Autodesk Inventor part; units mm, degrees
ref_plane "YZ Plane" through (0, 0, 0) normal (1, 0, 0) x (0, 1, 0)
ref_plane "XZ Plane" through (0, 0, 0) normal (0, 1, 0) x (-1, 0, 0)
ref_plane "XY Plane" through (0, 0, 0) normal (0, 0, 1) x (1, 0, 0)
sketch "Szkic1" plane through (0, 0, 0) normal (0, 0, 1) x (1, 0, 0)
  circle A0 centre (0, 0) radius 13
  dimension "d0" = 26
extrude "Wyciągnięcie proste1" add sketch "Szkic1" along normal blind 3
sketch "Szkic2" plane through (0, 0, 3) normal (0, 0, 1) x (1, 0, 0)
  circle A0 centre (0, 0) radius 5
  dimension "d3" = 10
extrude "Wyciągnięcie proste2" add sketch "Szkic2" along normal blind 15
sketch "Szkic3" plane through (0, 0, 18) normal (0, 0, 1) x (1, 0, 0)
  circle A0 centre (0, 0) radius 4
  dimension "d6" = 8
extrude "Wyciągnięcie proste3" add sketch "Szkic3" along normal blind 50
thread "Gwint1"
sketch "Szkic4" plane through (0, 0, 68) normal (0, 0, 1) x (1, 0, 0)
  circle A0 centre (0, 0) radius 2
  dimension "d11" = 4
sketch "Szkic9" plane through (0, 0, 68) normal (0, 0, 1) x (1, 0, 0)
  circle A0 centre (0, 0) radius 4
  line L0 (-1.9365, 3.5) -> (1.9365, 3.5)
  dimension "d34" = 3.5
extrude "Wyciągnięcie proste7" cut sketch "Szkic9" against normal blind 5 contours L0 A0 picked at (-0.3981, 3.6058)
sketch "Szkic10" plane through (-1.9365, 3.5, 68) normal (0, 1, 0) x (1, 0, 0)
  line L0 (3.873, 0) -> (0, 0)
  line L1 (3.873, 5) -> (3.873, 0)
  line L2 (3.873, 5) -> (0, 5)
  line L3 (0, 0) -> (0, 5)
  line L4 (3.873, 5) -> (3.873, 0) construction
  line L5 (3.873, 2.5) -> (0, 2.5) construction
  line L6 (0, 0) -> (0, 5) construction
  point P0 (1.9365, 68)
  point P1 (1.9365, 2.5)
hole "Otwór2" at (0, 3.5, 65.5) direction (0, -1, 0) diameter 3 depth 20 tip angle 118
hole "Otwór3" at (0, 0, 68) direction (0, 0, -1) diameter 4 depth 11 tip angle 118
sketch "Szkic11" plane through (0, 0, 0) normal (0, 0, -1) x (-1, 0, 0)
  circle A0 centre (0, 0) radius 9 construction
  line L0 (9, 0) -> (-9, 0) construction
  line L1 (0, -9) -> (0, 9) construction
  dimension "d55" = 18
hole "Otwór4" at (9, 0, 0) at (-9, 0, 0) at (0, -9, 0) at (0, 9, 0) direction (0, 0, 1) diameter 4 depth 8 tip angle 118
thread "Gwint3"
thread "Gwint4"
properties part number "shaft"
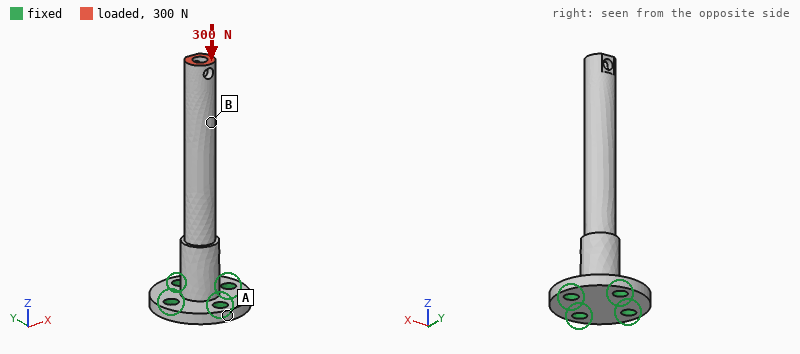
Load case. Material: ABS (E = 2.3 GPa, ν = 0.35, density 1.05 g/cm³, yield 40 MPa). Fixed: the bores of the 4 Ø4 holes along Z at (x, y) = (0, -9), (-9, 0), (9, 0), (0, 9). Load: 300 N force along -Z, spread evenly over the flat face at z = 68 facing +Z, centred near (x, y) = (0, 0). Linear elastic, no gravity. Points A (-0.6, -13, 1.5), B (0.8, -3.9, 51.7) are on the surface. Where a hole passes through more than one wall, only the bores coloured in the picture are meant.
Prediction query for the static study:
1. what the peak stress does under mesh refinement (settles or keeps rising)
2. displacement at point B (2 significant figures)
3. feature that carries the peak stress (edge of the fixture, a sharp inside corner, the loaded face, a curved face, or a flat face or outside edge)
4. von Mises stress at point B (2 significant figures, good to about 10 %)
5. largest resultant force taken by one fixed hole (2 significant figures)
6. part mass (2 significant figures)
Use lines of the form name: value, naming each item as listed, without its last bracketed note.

what the peak stress does under mesh refinement: keeps rising
displacement at point B: 0.17 mm
feature that carries the peak stress: a sharp inside corner
von Mises stress at point B: 6.9 MPa
largest resultant force taken by one fixed hole: 82 N
part mass: 5.2 g
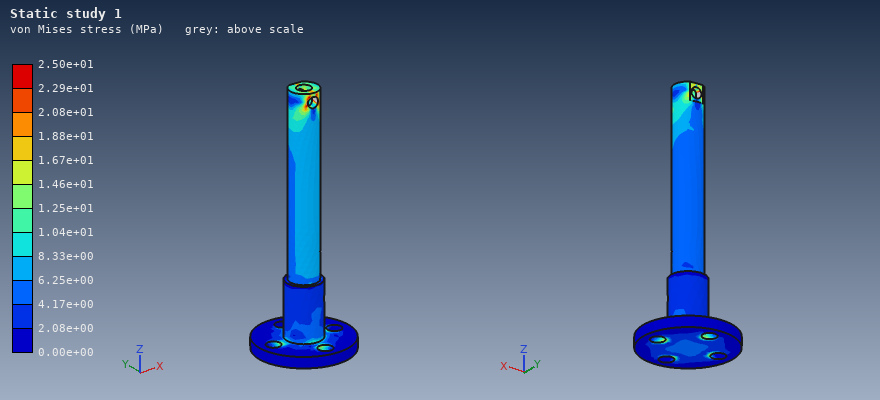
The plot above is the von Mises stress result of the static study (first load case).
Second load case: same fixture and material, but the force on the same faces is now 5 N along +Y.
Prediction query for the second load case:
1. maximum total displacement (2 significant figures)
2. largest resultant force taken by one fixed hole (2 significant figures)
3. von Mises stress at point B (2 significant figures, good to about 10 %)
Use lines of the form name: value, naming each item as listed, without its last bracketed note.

maximum total displacement: 0.78 mm
largest resultant force taken by one fixed hole: 23 N
von Mises stress at point B: 1.6 MPa
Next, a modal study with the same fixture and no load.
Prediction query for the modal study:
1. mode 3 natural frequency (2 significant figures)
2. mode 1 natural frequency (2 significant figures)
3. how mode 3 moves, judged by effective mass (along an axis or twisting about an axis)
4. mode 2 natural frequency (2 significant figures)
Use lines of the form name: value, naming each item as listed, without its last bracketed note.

mode 3 natural frequency: 2500 Hz
mode 1 natural frequency: 500 Hz
how mode 3 moves, judged by effective mass: along X
mode 2 natural frequency: 500 Hz
